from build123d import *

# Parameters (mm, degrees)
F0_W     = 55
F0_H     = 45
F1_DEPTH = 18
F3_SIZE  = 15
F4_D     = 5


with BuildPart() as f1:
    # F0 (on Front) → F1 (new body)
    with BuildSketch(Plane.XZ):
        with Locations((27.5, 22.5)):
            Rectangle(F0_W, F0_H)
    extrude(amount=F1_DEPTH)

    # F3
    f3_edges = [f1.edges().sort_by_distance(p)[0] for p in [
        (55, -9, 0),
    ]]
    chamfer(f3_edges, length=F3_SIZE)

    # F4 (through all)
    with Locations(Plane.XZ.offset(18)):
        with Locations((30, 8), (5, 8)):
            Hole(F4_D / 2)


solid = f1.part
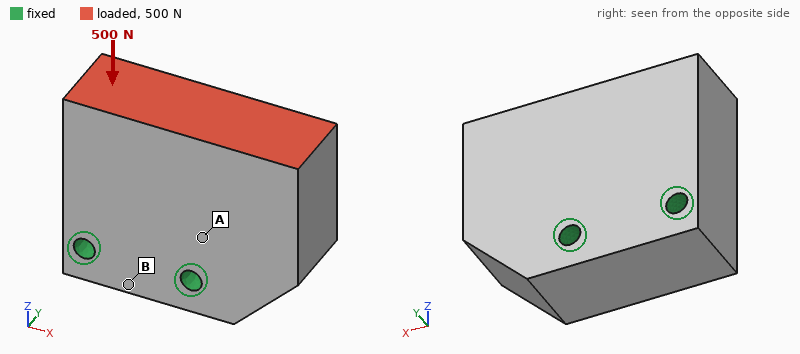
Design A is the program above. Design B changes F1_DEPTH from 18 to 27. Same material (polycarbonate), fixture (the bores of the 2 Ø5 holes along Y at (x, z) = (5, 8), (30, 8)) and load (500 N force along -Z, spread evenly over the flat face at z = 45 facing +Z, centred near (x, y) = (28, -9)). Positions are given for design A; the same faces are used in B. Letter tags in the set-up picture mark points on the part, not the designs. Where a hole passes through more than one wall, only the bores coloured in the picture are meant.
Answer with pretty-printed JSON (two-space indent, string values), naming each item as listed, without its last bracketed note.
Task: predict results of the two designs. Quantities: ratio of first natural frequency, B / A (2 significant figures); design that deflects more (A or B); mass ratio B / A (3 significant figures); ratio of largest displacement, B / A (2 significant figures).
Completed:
{
  "ratio of first natural frequency, B / A": "1.3",
  "design that deflects more": "A",
  "mass ratio B / A": "1.50",
  "ratio of largest displacement, B / A": "0.66"
}
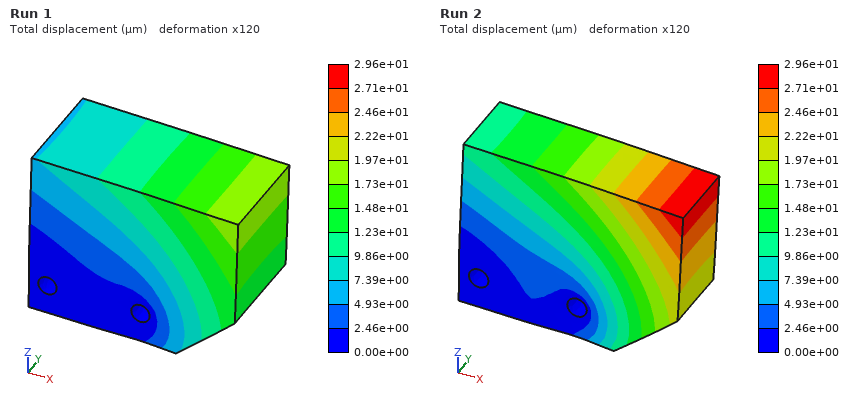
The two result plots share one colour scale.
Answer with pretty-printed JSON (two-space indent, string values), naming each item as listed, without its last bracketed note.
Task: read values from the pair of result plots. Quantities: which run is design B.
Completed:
{
  "which run is design B": "Run 1"
}
